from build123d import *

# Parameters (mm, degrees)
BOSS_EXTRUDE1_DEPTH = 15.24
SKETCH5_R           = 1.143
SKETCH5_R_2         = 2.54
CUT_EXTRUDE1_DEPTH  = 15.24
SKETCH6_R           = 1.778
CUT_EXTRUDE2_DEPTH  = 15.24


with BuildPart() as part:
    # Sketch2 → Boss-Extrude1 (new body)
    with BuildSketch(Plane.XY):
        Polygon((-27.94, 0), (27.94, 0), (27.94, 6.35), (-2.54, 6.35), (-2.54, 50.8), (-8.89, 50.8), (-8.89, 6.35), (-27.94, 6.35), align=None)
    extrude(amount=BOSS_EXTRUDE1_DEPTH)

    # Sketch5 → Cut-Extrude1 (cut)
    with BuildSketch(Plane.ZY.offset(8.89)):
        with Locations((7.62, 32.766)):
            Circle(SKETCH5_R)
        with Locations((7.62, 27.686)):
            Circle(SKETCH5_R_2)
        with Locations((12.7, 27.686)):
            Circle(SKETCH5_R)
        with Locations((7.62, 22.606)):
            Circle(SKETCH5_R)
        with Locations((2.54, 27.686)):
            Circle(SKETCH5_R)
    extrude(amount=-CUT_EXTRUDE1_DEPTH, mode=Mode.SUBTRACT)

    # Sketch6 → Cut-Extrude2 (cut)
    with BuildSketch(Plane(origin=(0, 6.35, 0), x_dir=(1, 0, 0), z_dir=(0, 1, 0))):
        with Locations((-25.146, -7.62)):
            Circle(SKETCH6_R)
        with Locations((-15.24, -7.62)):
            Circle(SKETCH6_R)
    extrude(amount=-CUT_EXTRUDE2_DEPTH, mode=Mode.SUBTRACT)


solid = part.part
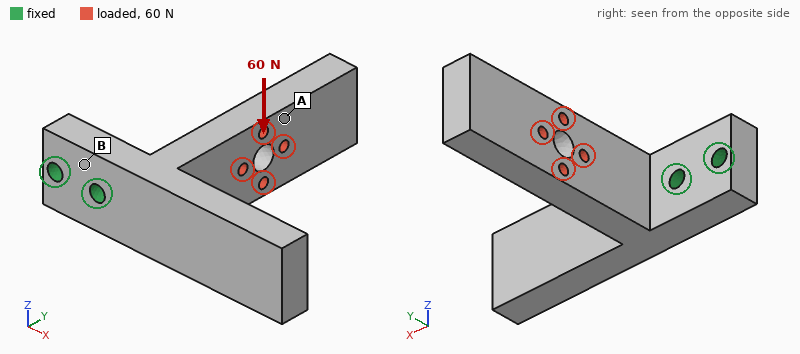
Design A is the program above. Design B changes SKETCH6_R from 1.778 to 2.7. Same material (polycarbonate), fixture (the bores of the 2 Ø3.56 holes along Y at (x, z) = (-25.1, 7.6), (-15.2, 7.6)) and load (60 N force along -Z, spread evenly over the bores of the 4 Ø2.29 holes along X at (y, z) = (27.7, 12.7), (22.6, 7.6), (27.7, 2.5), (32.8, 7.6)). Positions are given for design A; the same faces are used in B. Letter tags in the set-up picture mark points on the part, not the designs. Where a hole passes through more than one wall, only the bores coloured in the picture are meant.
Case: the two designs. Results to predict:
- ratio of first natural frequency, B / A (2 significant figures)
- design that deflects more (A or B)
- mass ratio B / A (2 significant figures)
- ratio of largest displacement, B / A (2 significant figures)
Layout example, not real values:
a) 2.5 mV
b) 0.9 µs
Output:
a) 1.0
b) A
c) 0.98
d) 0.83
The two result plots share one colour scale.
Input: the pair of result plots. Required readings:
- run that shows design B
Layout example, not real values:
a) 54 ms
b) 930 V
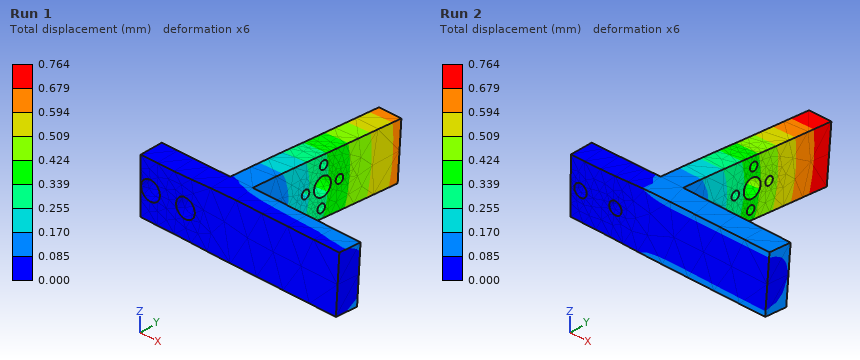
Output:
a) Run 1
